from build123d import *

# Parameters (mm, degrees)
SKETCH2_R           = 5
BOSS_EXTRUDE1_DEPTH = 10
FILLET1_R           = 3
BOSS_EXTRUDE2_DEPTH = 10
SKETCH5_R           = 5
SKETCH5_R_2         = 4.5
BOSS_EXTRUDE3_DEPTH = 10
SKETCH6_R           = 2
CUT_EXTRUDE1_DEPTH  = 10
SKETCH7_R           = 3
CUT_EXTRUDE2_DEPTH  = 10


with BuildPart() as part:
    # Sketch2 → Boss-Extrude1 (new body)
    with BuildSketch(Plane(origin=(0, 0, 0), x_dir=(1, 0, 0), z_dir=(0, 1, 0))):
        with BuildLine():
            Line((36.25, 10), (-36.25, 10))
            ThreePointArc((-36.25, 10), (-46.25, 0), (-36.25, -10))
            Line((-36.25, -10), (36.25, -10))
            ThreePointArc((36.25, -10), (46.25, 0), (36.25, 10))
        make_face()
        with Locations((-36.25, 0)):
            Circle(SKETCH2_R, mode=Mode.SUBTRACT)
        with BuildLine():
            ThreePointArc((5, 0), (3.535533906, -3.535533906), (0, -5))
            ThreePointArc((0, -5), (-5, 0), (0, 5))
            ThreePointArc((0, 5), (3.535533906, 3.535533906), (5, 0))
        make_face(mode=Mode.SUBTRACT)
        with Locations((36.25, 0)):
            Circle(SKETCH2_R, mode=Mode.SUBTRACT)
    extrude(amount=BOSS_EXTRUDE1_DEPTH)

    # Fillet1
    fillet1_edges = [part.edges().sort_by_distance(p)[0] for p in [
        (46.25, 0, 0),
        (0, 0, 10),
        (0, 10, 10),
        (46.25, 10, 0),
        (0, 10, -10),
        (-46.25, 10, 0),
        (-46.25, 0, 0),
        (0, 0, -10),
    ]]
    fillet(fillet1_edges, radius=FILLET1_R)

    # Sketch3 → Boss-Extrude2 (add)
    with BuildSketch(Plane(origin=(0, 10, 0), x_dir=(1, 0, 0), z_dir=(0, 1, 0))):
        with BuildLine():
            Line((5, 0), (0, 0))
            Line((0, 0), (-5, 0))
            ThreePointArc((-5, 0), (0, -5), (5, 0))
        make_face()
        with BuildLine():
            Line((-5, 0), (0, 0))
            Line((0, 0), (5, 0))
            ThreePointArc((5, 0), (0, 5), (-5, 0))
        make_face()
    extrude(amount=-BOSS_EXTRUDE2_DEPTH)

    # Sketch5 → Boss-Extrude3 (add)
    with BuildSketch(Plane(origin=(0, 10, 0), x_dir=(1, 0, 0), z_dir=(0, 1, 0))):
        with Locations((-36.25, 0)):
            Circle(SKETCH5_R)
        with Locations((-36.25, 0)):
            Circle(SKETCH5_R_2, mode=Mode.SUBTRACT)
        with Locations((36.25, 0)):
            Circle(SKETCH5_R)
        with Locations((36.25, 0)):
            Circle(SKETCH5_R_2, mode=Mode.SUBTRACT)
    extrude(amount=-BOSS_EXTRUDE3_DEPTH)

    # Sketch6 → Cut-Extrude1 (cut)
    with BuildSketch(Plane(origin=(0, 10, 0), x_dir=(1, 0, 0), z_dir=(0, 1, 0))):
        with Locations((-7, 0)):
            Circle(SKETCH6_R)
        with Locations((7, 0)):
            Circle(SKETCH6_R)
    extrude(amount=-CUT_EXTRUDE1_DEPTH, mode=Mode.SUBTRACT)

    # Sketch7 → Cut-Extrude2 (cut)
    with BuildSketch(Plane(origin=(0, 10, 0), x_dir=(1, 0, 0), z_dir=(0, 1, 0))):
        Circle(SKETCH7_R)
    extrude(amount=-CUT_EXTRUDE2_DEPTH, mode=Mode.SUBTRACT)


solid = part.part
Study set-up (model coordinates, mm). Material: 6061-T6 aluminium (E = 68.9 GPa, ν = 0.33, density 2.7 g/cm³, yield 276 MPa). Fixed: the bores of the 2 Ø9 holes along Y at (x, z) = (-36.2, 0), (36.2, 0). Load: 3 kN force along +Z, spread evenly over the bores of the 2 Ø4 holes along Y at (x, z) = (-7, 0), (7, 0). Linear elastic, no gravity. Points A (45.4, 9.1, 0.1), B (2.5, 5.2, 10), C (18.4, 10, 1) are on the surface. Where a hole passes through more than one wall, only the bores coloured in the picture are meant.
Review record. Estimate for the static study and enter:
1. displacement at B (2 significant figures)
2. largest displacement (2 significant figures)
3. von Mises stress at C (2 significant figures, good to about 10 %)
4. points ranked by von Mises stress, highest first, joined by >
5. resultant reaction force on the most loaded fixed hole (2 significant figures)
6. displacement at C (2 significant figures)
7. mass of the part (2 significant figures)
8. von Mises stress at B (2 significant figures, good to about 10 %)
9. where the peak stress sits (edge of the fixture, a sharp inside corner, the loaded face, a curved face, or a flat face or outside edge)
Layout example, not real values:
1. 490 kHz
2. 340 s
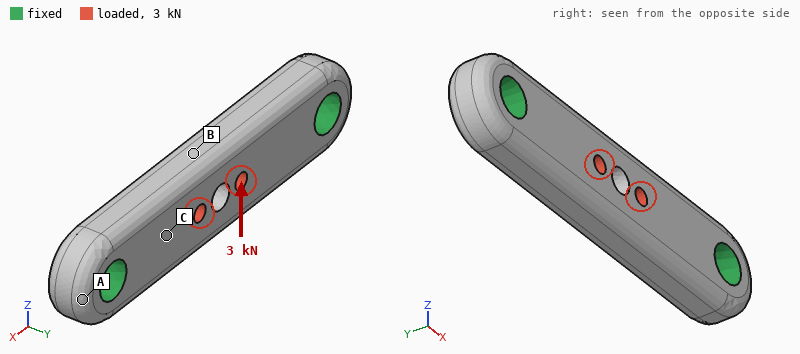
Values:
1. 24 µm
2. 25 µm
3. 21 MPa
4. B > C > A
5. 1.5 kN
6. 13 µm
7. 41 g
8. 38 MPa
9. edge of the fixture
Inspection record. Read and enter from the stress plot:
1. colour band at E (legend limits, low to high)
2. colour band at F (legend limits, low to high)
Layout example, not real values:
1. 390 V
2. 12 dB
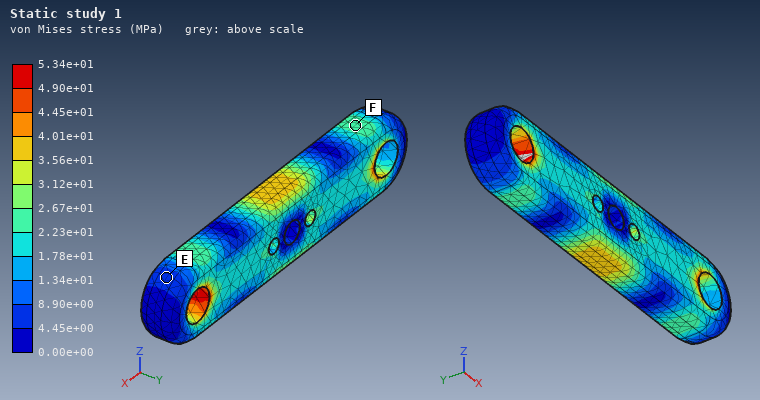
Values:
1. 4.45e+00 to 8.90e+00 MPa
2. 2.23e+01 to 2.67e+01 MPa
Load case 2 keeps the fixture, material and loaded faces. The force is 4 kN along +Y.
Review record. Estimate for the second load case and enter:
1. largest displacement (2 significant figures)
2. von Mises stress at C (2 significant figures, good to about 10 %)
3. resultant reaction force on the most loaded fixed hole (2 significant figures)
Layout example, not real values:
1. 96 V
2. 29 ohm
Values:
1. 72 µm
2. 13 MPa
3. 2.0 kN
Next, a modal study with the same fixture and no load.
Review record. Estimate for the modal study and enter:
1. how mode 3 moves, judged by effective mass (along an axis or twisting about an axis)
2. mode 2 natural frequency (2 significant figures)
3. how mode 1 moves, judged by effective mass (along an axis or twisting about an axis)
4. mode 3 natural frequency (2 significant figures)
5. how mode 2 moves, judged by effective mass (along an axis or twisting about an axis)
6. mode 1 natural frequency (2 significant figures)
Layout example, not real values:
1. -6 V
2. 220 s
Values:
1. twisting about X
2. 14 kHz
3. along Y
4. 18 kHz
5. along Z
6. 10 kHz
